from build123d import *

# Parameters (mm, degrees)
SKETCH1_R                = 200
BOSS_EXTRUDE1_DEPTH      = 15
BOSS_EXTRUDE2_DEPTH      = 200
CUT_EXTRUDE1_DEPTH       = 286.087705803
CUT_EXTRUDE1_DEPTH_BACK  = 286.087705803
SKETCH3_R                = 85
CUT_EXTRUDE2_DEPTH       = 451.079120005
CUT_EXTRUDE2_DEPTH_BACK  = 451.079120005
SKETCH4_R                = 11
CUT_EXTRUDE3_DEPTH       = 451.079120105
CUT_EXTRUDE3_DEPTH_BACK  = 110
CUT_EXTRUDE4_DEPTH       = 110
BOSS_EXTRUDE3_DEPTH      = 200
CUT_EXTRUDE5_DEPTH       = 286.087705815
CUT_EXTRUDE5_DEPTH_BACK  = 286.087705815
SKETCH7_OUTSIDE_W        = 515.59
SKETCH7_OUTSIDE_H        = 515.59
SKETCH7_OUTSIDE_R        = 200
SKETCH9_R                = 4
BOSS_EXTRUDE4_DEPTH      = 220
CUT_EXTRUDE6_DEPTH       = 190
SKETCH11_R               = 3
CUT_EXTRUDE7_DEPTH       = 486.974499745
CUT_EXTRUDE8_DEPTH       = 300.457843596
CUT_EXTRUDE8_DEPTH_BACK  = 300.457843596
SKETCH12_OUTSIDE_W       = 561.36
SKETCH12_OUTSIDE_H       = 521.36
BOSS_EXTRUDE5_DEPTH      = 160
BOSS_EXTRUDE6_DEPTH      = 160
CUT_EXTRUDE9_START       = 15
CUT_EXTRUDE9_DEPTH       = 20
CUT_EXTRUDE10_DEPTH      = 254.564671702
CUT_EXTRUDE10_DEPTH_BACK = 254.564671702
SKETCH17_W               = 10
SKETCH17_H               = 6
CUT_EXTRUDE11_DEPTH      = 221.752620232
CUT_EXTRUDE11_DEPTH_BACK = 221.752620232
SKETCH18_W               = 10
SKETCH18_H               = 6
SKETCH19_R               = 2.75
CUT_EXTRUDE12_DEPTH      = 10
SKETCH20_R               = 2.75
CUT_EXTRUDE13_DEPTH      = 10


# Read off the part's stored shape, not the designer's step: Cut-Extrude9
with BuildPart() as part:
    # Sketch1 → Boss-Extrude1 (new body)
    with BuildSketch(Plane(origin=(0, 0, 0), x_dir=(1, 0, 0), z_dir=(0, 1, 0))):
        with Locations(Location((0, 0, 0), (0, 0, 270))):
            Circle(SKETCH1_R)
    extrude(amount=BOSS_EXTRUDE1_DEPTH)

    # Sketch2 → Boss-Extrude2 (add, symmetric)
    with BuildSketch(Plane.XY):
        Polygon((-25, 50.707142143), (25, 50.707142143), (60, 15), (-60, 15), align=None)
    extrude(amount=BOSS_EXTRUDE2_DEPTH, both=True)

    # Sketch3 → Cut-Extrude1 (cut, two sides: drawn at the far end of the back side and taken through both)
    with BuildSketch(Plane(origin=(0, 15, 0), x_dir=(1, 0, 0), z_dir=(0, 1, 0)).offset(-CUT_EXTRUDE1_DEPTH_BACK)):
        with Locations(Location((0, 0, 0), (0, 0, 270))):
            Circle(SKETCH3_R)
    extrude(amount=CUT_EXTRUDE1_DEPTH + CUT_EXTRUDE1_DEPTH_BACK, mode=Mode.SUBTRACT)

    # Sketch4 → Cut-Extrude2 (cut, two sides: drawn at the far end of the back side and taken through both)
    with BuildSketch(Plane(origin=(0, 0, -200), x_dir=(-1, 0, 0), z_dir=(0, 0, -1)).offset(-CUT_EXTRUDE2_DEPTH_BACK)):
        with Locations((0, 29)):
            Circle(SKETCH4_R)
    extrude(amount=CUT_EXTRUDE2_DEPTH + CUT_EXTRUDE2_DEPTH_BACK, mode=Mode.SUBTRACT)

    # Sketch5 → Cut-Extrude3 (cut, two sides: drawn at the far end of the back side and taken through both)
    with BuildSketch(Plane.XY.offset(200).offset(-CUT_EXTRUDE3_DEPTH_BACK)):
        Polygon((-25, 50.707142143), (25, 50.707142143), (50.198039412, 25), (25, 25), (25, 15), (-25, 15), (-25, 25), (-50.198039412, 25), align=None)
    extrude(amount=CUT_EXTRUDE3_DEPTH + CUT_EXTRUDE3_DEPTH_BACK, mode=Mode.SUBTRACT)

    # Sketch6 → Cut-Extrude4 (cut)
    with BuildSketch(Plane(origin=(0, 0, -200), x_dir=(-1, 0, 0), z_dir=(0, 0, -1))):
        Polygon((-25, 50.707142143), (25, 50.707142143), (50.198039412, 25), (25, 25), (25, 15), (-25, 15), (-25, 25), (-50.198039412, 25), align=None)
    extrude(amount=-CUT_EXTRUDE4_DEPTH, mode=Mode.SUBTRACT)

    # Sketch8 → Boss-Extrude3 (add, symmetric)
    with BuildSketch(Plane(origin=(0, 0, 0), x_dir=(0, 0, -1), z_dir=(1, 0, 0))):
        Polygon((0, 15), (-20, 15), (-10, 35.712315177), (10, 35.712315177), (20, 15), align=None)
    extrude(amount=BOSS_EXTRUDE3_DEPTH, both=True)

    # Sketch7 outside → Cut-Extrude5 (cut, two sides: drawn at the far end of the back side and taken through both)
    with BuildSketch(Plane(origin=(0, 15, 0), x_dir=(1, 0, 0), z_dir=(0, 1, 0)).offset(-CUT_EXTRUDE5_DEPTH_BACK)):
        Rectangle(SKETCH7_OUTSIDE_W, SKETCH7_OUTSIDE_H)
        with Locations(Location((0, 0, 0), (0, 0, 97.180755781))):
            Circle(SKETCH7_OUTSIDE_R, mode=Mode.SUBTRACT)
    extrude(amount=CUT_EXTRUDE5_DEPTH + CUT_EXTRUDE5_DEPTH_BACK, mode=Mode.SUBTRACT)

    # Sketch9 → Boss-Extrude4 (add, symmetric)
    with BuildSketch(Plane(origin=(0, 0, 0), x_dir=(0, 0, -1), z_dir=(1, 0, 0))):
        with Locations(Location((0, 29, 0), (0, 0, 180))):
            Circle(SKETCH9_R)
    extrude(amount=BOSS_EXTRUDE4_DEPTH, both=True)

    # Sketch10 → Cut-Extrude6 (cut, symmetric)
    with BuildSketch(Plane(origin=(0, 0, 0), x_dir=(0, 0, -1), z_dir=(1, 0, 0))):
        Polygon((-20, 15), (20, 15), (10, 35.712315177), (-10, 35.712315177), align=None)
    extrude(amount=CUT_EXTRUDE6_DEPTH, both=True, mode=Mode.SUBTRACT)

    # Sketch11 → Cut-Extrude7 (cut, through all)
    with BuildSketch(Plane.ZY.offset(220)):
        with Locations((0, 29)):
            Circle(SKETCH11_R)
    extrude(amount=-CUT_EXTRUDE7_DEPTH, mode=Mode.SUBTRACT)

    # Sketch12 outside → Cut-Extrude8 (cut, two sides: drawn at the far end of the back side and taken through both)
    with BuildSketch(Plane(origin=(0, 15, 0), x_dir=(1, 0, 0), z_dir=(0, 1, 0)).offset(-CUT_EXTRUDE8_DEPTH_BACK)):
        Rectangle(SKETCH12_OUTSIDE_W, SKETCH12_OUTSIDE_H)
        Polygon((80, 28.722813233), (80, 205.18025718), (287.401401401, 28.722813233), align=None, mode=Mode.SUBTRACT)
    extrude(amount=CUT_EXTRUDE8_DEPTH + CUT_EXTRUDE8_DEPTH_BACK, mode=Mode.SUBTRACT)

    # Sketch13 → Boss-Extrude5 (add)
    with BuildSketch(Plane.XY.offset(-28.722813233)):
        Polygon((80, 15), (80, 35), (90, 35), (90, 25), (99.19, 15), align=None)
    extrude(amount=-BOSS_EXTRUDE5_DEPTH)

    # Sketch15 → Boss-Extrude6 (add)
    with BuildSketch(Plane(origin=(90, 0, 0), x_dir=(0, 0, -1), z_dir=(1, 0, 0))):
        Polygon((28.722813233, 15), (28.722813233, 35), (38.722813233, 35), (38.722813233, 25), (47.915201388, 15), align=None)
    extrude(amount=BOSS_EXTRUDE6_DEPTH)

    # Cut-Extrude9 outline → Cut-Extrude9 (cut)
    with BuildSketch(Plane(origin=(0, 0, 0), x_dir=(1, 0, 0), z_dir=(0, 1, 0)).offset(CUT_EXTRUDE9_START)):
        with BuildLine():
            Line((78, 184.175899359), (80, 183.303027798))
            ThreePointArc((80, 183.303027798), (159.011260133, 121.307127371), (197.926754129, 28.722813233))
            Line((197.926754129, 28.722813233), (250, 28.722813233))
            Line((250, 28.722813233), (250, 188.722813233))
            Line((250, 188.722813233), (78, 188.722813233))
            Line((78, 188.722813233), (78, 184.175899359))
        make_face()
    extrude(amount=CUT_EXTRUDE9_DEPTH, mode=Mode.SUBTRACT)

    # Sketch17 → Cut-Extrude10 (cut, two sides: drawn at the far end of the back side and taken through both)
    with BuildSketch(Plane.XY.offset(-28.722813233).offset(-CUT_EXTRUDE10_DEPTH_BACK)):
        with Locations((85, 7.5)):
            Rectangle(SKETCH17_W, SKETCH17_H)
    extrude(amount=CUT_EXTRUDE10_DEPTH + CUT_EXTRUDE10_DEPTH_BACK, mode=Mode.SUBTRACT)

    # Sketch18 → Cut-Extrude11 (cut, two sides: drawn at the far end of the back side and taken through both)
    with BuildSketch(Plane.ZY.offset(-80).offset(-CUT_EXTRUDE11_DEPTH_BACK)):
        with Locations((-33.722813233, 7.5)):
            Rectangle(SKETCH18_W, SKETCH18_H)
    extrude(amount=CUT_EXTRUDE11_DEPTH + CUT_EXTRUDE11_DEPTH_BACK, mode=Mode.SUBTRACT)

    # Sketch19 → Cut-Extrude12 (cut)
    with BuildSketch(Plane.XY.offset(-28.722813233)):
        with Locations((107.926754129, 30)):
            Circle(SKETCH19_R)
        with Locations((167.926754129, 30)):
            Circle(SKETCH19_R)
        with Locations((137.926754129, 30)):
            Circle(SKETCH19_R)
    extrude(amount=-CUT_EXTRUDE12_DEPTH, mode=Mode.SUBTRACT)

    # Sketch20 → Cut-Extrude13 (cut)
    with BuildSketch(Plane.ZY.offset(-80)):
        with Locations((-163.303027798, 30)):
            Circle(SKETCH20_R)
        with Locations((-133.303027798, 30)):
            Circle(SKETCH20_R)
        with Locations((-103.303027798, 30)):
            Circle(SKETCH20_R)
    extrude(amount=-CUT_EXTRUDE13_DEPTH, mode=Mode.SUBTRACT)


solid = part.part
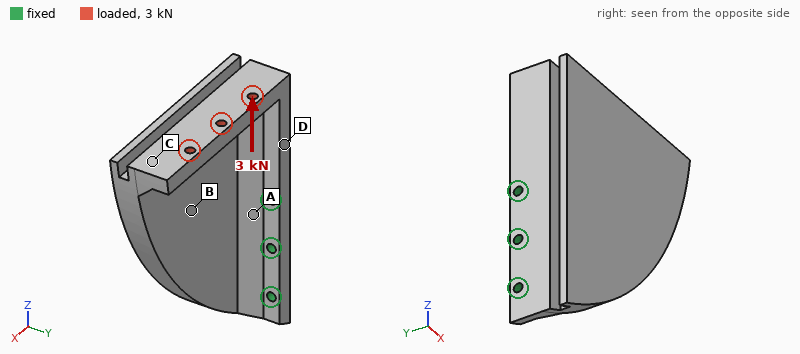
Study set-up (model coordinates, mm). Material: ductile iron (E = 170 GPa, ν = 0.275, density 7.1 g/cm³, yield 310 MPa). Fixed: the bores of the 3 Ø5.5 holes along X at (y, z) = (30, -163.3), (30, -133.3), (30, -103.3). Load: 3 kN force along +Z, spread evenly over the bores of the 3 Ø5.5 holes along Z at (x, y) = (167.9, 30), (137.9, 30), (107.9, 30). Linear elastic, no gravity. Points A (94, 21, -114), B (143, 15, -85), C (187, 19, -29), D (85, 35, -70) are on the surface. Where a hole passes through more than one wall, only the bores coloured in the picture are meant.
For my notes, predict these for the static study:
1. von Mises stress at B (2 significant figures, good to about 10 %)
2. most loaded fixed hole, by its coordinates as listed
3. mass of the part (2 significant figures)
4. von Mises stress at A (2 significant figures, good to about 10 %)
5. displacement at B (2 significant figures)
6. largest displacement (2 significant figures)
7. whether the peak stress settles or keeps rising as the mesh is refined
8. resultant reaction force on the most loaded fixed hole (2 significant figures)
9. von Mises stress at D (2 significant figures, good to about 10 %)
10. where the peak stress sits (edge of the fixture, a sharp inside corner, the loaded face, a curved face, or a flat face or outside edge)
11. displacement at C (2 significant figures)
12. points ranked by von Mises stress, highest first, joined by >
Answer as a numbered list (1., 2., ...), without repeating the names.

1. 13 MPa
2. (30, -103.3)
3. 1.6 kg
4. 26 MPa
5. 0.038 mm
6. 0.12 mm
7. keeps rising
8. 3.4 kN
9. 19 MPa
10. edge of the fixture
11. 0.11 mm
12. A > D > B > C
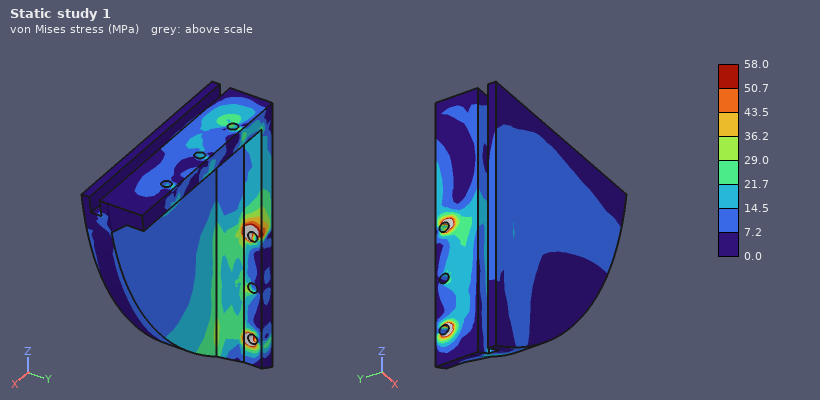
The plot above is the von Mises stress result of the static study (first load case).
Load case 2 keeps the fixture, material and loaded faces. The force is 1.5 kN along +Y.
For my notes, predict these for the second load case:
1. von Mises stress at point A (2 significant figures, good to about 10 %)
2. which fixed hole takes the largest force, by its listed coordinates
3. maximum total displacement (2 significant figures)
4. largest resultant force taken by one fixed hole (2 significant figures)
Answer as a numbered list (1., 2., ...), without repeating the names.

1. 34 MPa
2. (30, -103.3)
3. 0.27 mm
4. 3.8 kN
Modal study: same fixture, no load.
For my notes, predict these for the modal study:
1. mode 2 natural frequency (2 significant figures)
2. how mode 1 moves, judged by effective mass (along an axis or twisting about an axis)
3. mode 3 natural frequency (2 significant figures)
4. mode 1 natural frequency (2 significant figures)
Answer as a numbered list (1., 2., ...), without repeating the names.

1. 1200 Hz
2. along Y
3. 2000 Hz
4. 500 Hz
